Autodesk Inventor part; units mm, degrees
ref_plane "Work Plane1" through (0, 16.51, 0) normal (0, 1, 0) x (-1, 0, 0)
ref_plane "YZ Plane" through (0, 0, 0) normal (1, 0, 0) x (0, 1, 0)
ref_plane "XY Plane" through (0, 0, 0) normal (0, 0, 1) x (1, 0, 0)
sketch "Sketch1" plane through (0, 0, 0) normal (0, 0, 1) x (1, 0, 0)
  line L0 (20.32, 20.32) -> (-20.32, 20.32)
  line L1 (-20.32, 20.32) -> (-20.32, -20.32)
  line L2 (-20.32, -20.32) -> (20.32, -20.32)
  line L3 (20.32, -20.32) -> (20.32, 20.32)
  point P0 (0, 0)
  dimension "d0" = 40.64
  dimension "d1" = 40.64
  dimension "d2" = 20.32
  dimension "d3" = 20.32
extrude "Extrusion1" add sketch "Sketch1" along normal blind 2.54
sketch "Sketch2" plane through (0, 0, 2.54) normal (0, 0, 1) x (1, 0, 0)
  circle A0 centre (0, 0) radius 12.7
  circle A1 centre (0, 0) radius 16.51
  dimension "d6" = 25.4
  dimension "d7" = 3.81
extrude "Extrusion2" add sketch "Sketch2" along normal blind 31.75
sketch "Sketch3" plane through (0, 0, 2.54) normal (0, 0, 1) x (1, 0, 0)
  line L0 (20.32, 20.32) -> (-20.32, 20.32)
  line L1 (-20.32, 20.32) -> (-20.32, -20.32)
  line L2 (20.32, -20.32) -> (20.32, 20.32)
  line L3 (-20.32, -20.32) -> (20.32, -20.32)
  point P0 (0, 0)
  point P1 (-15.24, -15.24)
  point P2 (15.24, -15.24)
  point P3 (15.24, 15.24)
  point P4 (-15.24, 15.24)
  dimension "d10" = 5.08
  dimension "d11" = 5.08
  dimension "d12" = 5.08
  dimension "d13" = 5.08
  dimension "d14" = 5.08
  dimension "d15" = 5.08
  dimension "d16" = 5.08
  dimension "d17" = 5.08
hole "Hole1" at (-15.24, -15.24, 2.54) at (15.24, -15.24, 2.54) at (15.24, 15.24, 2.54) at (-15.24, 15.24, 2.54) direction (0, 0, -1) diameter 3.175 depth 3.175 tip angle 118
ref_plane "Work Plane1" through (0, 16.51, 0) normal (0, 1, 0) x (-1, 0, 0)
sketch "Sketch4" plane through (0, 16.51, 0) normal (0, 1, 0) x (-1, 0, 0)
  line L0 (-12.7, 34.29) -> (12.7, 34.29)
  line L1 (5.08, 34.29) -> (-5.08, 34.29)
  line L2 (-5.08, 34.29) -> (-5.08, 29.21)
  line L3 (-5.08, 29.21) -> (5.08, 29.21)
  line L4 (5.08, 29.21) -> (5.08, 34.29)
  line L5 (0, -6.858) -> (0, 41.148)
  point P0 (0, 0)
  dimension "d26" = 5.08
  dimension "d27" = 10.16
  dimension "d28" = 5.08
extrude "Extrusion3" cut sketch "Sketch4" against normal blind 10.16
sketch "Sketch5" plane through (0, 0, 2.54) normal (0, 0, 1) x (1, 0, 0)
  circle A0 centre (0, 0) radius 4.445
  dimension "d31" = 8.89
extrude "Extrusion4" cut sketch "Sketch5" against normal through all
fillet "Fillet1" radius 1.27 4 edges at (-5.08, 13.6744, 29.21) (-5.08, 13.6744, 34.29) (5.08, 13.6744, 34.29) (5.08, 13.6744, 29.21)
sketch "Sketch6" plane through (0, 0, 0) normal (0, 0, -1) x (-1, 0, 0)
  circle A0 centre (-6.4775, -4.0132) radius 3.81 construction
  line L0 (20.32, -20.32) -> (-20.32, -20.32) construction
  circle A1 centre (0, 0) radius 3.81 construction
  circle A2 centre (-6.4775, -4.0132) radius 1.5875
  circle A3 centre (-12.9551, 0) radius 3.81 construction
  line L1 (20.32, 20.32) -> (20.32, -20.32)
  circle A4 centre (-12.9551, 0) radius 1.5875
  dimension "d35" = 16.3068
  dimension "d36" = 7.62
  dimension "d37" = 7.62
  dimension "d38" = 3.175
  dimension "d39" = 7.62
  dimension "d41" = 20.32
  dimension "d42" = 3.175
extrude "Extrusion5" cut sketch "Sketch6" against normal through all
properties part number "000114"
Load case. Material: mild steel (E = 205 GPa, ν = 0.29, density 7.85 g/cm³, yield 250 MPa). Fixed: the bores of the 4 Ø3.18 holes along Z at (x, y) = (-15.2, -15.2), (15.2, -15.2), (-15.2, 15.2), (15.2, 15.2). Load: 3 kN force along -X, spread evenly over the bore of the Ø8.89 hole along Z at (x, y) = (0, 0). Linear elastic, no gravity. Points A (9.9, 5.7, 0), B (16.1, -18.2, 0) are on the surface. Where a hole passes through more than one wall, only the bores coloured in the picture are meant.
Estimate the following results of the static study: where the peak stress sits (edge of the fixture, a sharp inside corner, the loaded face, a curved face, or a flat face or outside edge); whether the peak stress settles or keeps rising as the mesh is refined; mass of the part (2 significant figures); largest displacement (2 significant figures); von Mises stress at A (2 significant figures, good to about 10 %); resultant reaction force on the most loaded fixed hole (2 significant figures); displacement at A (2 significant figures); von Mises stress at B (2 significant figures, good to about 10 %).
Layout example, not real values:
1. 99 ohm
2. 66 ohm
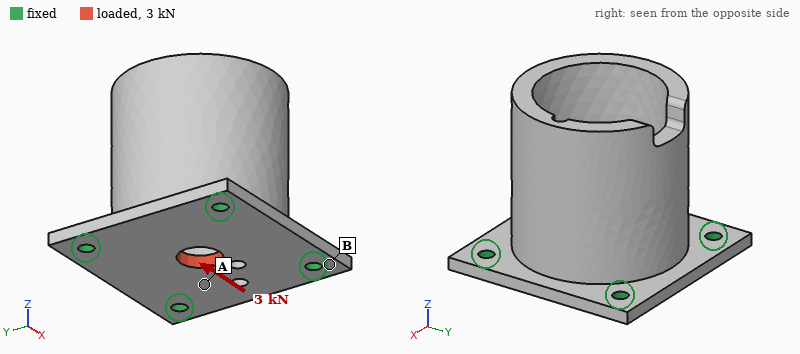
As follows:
1. a sharp inside corner
2. keeps rising
3. 120 g
4. 4.3 µm
5. 25 MPa
6. 820 N
7. 2.2 µm
8. 13 MPa
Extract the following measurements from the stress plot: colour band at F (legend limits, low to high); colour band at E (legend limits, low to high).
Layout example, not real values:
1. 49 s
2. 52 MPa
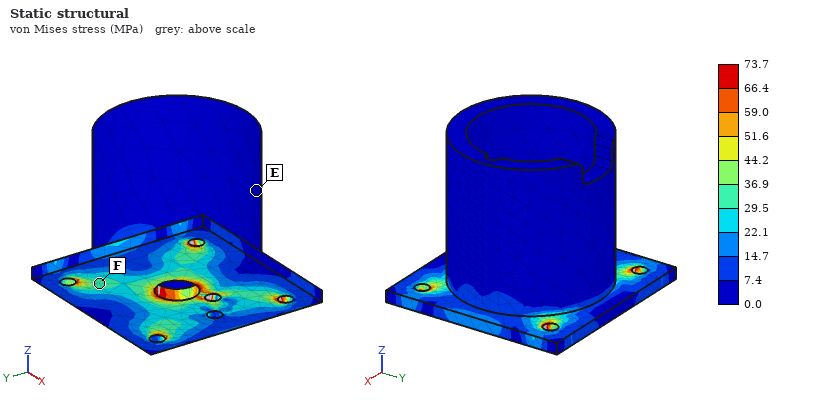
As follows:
1. 29.5 to 36.9 MPa
2. 0.0 to 7.4 MPa
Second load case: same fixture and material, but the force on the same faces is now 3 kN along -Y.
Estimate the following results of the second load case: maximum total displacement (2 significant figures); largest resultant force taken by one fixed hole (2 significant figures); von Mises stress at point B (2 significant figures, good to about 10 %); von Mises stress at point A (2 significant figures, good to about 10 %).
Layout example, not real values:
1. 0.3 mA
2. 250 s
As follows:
1. 3.9 µm
2. 830 N
3. 13 MPa
4. 24 MPa
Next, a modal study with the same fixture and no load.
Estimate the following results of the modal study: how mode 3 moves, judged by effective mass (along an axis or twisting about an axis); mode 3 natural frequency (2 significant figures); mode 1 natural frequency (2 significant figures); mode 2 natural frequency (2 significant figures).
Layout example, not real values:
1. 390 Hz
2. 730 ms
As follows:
1. along Z
2. 9800 Hz
3. 6300 Hz
4. 6300 Hz
